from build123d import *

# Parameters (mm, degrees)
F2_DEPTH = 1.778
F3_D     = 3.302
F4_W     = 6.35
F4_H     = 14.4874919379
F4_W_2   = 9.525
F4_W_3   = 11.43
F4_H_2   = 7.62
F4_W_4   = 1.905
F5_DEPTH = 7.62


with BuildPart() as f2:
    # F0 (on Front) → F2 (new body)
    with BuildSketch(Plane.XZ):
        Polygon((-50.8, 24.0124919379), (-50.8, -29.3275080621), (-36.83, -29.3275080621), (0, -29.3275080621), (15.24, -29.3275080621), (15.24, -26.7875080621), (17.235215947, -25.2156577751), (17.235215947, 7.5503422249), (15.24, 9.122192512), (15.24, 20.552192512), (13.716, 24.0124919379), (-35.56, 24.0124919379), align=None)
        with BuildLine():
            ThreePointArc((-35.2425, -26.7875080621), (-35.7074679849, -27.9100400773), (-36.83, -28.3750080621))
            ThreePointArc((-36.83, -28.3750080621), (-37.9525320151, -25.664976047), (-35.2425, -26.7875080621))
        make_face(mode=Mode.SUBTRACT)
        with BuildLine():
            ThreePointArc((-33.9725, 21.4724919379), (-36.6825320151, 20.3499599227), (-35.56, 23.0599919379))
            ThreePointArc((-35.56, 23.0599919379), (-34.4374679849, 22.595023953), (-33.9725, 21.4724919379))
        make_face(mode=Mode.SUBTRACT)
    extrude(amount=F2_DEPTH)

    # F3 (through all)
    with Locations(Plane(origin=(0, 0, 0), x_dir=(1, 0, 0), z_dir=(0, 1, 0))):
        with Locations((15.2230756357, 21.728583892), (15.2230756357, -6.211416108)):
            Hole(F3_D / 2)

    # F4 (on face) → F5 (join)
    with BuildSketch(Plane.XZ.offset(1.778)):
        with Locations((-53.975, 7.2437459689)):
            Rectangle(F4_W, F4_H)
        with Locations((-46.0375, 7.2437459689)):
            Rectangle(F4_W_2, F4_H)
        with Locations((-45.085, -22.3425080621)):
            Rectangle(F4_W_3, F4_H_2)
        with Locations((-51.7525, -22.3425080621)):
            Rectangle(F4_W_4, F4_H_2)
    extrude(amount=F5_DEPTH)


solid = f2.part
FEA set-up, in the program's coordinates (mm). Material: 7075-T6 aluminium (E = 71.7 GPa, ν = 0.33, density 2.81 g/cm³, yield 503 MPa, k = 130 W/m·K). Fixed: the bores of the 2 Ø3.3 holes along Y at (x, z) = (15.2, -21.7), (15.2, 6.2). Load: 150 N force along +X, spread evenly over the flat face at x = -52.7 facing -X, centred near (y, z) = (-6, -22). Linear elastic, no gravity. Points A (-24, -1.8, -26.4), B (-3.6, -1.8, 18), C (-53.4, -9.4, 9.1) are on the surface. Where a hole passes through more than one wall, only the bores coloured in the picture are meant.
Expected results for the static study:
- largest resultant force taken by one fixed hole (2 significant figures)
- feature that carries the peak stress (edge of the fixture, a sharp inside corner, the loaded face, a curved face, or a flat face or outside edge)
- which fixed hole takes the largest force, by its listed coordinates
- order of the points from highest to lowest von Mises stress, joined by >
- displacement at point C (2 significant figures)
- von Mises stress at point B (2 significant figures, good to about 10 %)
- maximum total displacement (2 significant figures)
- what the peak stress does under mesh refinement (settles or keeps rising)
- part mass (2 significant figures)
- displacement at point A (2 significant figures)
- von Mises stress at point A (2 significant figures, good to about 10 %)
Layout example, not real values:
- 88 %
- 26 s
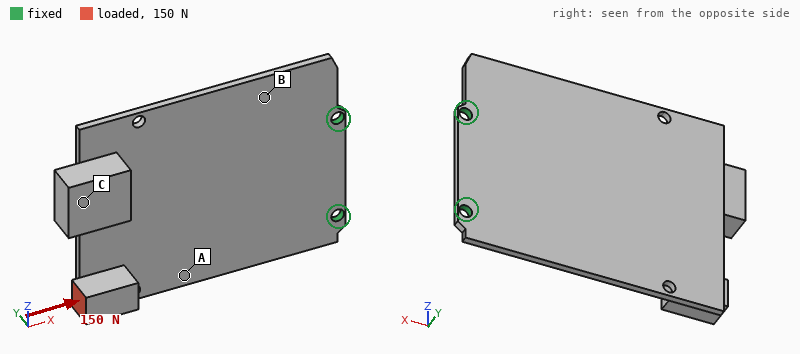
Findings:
- 150 N
- edge of the fixture
- (15.2, -21.7)
- A > B > C
- 0.94 mm
- 22 MPa
- 1.1 mm
- keeps rising
- 25 g
- 0.34 mm
- 36 MPa
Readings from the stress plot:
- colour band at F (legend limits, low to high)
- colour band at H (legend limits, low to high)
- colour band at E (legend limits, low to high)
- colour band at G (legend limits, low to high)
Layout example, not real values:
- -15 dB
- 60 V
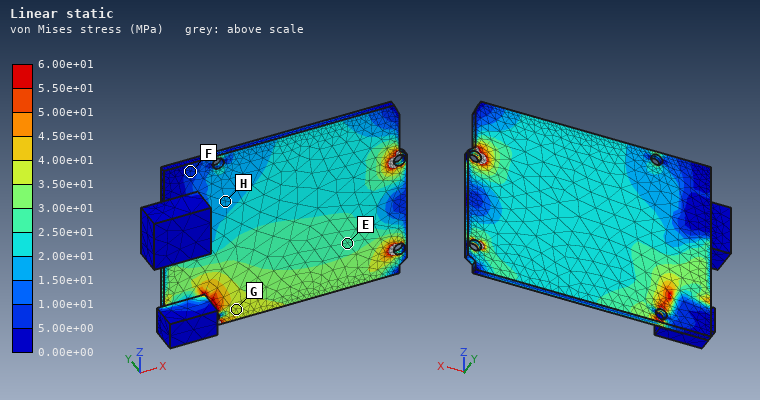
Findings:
- 5.00e+00 to 1.00e+01 MPa
- 1.50e+01 to 2.00e+01 MPa
- 2.50e+01 to 3.00e+01 MPa
- 3.50e+01 to 4.00e+01 MPa
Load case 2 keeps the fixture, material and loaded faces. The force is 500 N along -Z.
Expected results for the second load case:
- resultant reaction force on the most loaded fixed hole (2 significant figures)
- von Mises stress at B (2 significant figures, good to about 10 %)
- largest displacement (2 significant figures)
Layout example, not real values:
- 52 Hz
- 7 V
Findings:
- 1.2 kN
- 28 MPa
- 1.1 mm
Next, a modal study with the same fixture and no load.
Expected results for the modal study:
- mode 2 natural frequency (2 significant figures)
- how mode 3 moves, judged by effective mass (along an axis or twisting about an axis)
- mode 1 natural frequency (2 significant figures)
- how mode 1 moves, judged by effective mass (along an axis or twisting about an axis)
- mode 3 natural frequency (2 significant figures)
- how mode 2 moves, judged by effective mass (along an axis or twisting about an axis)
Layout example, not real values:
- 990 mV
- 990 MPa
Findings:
- 670 Hz
- along Y
- 200 Hz
- along Y
- 1500 Hz
- twisting about X
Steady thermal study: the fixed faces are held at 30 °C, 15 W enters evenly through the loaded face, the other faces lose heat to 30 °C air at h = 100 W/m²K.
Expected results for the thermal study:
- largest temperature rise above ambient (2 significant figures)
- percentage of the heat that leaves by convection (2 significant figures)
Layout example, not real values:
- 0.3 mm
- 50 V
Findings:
- 63 K
- 81 %
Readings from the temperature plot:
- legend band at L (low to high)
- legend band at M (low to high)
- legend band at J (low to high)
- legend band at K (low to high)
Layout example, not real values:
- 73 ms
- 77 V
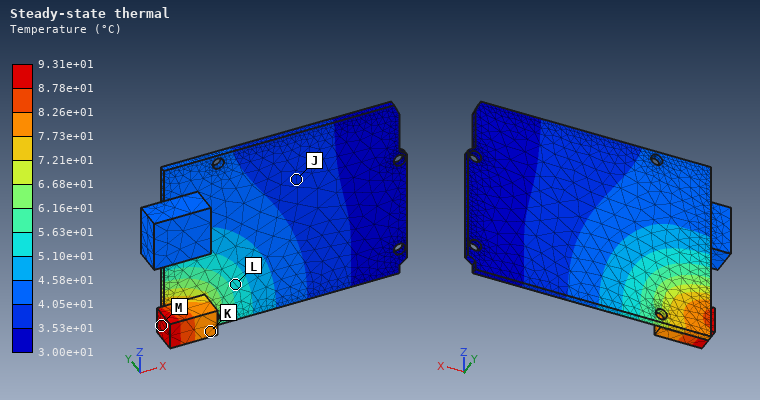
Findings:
- 5.10e+01 to 5.63e+01 °C
- 8.78e+01 to 9.31e+01 °C
- 3.53e+01 to 4.05e+01 °C
- 7.73e+01 to 8.26e+01 °C
